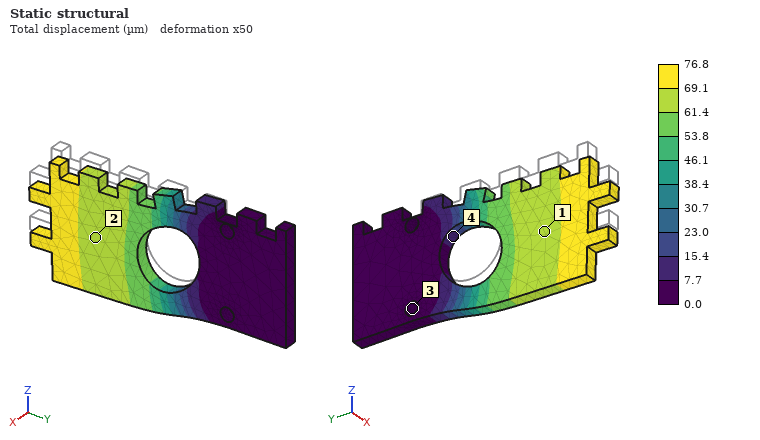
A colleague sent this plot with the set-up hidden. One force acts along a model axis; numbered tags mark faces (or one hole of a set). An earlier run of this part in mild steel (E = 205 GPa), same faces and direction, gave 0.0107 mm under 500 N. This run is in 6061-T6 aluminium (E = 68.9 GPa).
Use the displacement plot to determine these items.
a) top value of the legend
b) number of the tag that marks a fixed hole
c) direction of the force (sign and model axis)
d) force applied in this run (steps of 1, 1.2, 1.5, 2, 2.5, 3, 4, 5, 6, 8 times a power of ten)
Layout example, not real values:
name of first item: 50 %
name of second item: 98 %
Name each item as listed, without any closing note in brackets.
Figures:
top value of the legend: 76.8 µm
number of the tag that marks a fixed hole: 3
direction of the force: -Z
force applied in this run: 1.2 kN
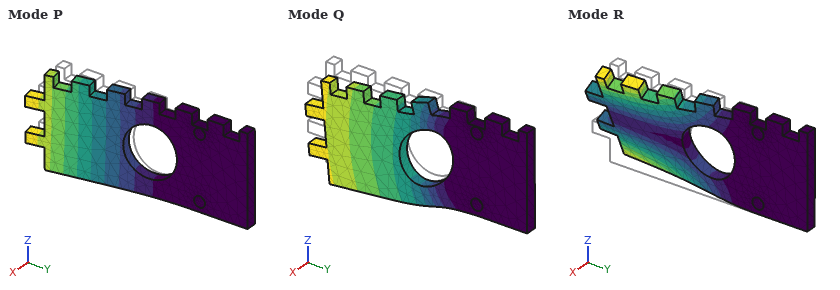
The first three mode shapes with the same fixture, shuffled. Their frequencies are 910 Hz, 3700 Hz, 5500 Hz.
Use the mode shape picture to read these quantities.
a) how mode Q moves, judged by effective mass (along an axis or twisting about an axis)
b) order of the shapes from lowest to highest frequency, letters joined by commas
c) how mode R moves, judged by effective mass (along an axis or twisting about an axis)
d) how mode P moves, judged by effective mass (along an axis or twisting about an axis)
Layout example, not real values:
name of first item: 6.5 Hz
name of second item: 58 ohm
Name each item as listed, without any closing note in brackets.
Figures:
how mode Q moves, judged by effective mass: along Z
order of the shapes from lowest to highest frequency, letters joined by commas: P, R, Q
how mode R moves, judged by effective mass: twisting about Y
how mode P moves, judged by effective mass: along X
